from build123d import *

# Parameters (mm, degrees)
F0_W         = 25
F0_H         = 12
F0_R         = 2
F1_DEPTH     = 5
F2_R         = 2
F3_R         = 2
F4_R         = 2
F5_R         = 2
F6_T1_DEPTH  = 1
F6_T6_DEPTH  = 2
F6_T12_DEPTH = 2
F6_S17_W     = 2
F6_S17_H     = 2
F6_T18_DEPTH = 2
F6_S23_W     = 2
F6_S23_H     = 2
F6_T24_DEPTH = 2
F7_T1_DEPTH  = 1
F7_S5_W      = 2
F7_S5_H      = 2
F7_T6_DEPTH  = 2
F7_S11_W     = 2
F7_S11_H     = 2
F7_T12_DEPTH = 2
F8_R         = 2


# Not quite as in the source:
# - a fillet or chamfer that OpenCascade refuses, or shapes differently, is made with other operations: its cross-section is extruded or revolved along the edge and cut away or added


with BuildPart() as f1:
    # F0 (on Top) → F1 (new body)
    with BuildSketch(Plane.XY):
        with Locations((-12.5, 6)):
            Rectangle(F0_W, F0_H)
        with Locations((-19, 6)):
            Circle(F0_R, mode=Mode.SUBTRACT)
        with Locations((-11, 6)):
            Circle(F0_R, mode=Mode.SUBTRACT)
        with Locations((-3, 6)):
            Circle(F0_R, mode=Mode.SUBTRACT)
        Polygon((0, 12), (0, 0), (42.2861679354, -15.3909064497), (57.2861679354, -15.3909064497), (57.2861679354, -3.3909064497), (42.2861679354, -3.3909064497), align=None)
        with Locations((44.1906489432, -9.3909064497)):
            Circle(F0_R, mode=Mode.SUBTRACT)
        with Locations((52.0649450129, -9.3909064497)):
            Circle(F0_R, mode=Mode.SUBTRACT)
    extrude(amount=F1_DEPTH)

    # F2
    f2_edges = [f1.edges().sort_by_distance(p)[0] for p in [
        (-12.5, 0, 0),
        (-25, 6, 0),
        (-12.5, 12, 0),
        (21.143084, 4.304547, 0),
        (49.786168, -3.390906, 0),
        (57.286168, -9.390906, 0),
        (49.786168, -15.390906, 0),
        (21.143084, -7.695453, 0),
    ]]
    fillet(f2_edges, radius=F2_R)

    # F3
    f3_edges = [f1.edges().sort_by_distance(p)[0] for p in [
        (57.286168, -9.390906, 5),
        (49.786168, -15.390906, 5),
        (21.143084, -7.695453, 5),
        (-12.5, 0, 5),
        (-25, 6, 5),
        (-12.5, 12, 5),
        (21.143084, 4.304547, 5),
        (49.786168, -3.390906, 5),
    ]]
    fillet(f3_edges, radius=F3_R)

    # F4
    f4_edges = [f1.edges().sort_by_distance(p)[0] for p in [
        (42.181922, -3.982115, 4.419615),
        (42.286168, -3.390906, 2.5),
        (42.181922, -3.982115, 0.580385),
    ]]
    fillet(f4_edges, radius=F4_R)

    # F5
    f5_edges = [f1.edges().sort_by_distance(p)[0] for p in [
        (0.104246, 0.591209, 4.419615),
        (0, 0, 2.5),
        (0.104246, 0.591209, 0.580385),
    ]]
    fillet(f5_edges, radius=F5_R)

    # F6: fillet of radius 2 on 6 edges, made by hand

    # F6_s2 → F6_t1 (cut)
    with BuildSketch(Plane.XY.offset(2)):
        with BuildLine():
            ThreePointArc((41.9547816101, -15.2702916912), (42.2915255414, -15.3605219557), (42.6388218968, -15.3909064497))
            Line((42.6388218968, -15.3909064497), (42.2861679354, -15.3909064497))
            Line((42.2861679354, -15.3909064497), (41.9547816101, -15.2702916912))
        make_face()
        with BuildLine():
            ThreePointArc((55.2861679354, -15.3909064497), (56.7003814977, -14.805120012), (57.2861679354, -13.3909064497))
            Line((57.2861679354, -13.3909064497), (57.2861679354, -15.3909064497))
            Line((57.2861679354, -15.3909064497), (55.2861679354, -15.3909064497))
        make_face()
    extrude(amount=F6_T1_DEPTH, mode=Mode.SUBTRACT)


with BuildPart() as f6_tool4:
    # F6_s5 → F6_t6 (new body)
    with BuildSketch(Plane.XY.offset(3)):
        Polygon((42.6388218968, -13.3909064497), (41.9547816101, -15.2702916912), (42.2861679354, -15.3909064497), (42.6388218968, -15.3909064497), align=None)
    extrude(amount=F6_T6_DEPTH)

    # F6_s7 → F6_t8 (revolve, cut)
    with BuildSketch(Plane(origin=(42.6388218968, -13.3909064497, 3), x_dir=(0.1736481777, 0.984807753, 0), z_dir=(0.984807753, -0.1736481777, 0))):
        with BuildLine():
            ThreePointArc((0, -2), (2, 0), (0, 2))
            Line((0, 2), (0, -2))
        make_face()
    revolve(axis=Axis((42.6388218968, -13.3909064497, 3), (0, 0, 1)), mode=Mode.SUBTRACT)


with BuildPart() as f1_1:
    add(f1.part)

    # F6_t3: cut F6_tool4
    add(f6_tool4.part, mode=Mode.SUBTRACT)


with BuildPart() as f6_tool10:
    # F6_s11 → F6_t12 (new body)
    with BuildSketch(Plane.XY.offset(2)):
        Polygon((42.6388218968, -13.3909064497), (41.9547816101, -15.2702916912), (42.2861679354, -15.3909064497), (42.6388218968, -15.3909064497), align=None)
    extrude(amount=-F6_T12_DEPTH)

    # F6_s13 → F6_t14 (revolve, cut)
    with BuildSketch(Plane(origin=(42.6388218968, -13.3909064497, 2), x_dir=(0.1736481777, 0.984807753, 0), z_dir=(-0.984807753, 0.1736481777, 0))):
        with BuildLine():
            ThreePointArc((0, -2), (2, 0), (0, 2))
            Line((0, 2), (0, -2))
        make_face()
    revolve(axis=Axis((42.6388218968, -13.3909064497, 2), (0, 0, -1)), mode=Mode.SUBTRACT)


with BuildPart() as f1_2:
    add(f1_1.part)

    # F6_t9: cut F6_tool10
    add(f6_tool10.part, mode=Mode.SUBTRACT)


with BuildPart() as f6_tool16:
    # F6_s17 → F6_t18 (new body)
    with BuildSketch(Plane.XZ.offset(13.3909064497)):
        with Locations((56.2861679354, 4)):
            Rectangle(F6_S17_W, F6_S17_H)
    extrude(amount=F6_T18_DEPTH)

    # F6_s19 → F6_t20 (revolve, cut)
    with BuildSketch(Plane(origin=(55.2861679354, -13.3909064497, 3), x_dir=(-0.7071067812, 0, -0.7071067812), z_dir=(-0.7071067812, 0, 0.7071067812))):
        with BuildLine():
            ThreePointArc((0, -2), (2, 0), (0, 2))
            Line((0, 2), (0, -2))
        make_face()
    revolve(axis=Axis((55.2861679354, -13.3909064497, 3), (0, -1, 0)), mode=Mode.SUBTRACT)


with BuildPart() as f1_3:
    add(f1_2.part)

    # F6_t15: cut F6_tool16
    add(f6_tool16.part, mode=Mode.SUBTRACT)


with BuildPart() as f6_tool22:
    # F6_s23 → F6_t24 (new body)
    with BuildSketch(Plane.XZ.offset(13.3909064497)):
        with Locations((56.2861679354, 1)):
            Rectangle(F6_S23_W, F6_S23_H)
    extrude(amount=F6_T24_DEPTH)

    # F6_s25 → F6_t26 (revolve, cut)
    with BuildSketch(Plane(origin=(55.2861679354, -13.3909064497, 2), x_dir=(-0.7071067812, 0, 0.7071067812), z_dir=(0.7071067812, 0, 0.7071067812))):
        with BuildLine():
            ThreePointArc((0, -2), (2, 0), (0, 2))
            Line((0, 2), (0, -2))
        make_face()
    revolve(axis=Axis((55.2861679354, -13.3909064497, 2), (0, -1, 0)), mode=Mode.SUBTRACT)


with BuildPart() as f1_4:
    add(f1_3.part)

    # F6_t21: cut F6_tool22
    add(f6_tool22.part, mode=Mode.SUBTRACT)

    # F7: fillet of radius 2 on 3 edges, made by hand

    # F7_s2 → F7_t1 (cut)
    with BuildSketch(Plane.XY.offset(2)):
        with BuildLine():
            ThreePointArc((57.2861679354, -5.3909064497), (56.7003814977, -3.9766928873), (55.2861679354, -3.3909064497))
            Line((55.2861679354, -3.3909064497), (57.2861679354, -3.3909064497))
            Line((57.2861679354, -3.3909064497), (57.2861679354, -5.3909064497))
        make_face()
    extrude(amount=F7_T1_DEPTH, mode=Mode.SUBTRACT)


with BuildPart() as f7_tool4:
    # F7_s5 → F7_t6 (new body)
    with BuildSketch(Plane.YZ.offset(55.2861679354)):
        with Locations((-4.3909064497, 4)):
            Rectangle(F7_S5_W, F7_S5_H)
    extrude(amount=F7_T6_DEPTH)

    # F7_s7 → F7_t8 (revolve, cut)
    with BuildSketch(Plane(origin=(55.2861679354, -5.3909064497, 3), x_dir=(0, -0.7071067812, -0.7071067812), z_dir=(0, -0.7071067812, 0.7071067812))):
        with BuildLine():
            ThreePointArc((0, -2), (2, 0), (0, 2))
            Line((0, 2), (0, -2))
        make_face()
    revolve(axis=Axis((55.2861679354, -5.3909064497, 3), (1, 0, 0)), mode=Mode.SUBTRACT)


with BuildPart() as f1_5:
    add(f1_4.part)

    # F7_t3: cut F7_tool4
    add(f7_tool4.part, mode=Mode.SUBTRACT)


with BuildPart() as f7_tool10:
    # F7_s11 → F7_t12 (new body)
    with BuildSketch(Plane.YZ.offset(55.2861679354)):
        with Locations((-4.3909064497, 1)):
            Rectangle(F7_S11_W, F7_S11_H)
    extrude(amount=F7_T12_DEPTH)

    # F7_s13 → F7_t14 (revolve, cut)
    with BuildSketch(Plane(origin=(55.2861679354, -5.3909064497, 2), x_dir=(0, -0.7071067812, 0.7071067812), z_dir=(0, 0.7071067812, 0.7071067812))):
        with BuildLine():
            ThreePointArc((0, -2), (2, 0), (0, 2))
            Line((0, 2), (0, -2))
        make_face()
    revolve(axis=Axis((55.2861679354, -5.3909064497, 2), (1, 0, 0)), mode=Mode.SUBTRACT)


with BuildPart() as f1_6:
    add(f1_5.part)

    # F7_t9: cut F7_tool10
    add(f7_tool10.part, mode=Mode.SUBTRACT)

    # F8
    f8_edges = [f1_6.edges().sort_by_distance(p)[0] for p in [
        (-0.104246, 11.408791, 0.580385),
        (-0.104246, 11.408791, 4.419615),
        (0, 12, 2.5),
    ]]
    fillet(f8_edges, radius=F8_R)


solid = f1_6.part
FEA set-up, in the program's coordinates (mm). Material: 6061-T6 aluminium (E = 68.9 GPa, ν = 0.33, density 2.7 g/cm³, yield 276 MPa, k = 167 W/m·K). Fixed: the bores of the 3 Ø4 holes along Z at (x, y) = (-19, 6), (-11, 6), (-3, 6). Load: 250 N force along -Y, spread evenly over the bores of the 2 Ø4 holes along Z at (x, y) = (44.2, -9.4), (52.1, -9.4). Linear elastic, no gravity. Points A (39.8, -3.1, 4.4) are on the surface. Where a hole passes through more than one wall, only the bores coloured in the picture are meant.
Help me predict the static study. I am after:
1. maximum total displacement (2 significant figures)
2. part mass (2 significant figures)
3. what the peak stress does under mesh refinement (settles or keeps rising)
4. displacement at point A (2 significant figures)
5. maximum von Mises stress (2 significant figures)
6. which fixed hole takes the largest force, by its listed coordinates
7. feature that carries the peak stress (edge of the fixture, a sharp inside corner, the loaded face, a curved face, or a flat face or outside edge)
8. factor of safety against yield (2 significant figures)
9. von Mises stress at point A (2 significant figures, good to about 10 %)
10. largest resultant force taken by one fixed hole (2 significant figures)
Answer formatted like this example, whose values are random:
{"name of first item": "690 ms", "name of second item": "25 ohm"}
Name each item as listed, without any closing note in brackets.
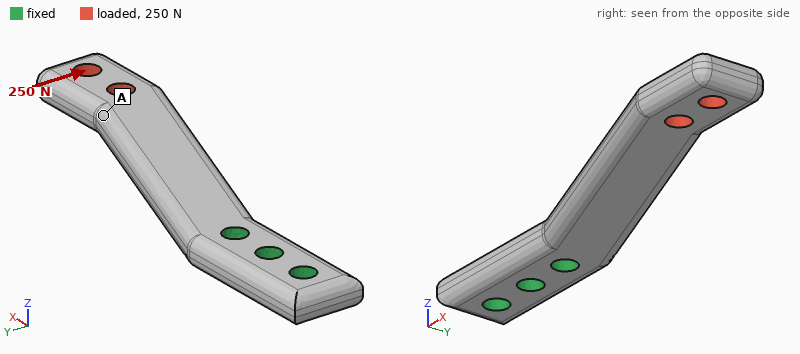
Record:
{"maximum total displacement": "0.50 mm", "part mass": "12 g", "what the peak stress does under mesh refinement": "settles", "displacement at point A": "0.29 mm", "maximum von Mises stress": "190 MPa", "which fixed hole takes the largest force, by its listed coordinates": "(-3, 6)", "feature that carries the peak stress": "a curved face", "factor of safety against yield": "1.5", "von Mises stress at point A": "28 MPa", "largest resultant force taken by one fixed hole": "820 N"}
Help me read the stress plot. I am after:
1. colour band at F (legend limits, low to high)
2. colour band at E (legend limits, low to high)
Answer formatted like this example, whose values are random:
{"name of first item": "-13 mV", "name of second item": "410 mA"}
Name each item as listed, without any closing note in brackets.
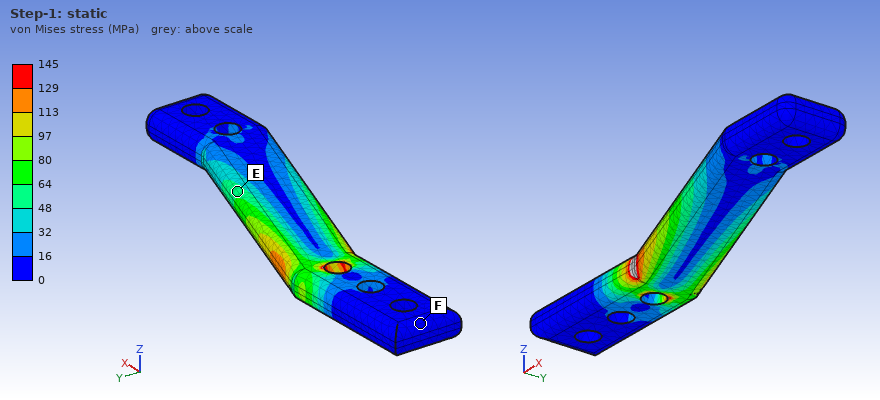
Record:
{"colour band at F": "0 to 16 MPa", "colour band at E": "48 to 64 MPa"}
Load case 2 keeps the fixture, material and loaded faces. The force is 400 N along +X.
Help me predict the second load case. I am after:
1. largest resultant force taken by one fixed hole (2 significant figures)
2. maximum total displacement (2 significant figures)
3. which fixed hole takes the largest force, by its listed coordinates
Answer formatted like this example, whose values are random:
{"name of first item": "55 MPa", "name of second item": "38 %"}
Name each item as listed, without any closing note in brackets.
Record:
{"largest resultant force taken by one fixed hole": "420 N", "maximum total displacement": "0.23 mm", "which fixed hole takes the largest force, by its listed coordinates": "(-3, 6)"}
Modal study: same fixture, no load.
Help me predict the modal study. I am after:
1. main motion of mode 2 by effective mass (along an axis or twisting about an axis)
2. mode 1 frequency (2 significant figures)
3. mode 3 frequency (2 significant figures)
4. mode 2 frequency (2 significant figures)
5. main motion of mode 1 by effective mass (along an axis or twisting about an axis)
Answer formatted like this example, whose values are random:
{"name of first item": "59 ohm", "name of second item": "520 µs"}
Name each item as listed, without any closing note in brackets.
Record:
{"main motion of mode 2 by effective mass": "along Y", "mode 1 frequency": "1100 Hz", "mode 3 frequency": "6300 Hz", "mode 2 frequency": "2200 Hz", "main motion of mode 1 by effective mass": "along Z"}
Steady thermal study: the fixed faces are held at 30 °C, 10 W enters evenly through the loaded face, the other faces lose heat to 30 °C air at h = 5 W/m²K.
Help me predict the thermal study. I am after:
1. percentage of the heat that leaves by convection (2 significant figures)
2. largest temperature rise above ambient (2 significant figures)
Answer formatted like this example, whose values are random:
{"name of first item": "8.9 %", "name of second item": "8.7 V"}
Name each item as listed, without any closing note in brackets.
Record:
{"percentage of the heat that leaves by convection": "3.0 %", "largest temperature rise above ambient": "61 K"}
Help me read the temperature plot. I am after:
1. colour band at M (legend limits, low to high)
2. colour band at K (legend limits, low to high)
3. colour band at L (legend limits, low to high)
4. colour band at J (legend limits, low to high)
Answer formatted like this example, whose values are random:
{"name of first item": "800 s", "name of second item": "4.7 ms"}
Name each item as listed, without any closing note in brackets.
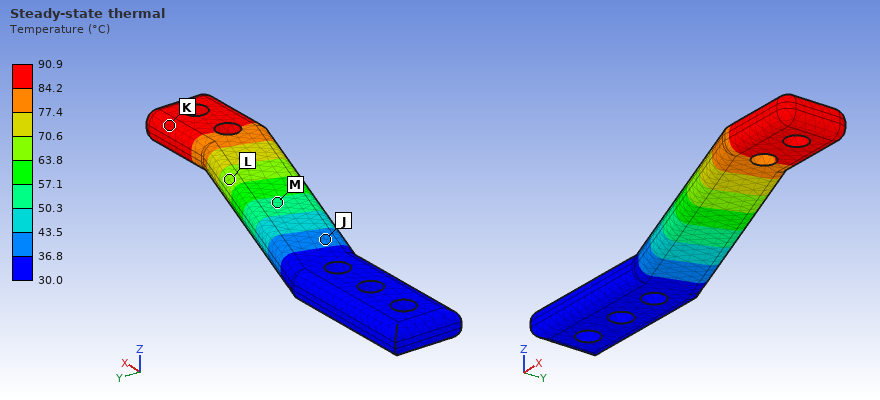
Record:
{"colour band at M": "50.3 to 57.1 °C", "colour band at K": "84.2 to 90.9 °C", "colour band at L": "63.8 to 70.6 °C", "colour band at J": "36.8 to 43.5 °C"}
